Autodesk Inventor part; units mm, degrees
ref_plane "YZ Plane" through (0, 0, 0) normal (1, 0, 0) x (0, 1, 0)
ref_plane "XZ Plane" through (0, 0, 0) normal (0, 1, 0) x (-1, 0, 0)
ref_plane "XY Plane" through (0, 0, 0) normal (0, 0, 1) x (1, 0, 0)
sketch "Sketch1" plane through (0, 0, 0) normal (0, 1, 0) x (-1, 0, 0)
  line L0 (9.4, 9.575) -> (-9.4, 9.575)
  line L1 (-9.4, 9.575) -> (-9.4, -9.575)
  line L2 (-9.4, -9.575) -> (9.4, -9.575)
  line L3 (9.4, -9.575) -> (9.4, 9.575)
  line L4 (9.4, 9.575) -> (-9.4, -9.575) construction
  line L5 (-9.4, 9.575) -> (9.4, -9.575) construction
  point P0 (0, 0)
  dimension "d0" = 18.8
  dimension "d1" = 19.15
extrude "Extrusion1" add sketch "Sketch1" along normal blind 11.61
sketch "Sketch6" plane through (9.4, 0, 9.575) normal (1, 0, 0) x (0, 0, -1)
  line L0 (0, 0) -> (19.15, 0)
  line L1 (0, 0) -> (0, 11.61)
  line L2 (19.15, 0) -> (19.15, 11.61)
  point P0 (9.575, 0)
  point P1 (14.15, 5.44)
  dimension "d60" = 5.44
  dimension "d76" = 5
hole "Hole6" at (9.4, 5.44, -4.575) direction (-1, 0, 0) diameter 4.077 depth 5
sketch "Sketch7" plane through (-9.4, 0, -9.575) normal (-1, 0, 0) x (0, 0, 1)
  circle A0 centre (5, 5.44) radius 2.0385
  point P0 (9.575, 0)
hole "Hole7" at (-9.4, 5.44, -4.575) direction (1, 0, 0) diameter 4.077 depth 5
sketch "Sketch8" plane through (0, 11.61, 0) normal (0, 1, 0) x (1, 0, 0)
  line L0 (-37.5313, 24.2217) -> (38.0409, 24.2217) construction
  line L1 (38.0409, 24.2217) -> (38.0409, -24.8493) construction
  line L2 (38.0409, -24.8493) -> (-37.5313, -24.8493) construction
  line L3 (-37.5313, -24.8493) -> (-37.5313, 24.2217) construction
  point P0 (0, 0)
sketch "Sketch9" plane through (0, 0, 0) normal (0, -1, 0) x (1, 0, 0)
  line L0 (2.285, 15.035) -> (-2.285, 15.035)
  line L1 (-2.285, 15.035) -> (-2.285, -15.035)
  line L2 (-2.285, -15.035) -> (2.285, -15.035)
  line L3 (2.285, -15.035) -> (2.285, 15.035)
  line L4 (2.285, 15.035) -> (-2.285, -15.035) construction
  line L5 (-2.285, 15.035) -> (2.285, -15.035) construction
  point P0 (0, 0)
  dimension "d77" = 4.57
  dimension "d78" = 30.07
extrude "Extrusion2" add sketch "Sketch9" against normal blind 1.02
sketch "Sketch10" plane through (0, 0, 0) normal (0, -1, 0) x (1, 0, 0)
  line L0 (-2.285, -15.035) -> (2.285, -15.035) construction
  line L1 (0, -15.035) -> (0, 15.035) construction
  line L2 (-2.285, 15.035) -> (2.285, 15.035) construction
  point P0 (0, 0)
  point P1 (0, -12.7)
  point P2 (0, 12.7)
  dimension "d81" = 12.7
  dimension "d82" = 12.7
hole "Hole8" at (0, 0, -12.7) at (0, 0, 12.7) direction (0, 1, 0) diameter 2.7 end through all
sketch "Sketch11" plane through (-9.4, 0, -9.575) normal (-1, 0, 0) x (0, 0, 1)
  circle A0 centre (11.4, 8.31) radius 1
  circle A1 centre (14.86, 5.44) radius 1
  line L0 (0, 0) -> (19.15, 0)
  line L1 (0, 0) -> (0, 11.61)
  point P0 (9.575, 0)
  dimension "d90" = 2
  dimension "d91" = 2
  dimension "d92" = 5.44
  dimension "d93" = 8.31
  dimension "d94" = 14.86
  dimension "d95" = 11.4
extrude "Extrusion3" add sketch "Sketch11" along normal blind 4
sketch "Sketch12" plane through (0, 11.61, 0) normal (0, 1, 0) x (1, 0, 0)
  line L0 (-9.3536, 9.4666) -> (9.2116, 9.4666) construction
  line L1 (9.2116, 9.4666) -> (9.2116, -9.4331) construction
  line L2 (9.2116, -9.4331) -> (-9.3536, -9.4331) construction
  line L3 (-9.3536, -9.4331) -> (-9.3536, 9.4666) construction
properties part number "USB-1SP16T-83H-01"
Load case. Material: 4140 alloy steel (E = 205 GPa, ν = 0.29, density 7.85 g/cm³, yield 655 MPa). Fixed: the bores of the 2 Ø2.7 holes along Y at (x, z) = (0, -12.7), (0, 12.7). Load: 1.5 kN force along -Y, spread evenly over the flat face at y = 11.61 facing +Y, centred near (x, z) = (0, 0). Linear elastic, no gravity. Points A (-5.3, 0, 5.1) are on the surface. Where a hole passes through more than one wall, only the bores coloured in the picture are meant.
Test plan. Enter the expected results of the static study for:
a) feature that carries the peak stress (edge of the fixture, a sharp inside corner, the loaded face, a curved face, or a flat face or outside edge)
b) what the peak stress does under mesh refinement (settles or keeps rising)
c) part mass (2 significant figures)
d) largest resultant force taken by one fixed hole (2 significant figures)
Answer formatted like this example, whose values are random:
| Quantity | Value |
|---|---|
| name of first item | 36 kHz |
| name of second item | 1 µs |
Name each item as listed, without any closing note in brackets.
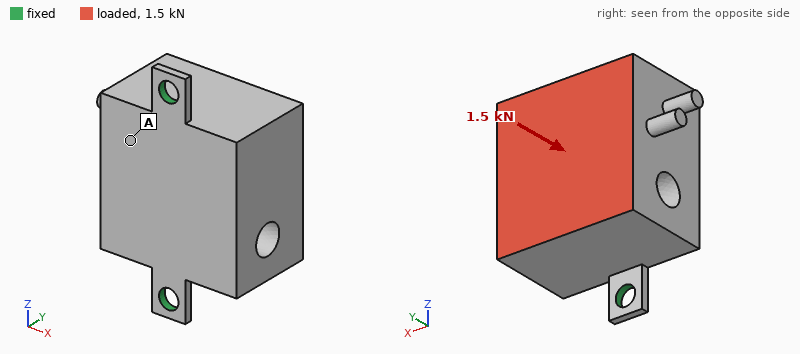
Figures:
| Quantity | Value |
|---|---|
| feature that carries the peak stress | edge of the fixture |
| what the peak stress does under mesh refinement | keeps rising |
| part mass | 32 g |
| largest resultant force taken by one fixed hole | 850 N |
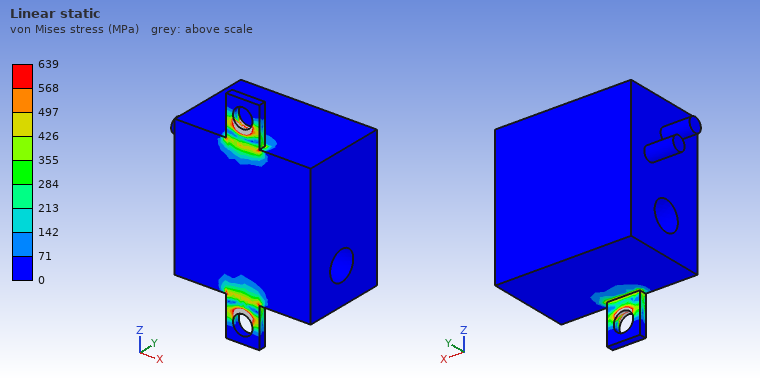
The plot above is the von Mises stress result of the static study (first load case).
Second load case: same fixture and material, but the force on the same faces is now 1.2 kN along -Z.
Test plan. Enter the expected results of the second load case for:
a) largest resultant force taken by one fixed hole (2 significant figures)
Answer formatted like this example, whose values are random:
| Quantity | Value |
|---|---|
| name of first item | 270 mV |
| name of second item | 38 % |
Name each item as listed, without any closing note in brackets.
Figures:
| Quantity | Value |
|---|---|
| largest resultant force taken by one fixed hole | 880 N |
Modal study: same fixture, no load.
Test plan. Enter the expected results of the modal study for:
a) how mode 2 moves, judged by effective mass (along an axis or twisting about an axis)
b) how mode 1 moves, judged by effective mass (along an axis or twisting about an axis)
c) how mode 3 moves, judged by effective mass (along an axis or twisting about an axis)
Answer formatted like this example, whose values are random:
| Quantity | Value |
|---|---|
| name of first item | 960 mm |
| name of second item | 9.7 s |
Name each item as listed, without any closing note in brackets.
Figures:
| Quantity | Value |
|---|---|
| how mode 2 moves, judged by effective mass | along Y |
| how mode 1 moves, judged by effective mass | along X |
| how mode 3 moves, judged by effective mass | along Z |
